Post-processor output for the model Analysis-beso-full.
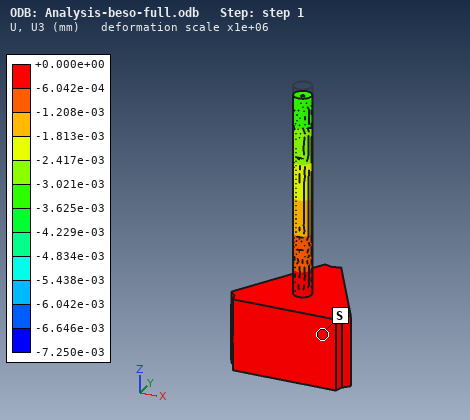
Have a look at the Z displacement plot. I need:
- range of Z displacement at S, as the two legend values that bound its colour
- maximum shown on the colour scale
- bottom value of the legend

-6.042e-04 to +0.000e+00 mm
+0.000e+00 mm
-7.250e-03 mm
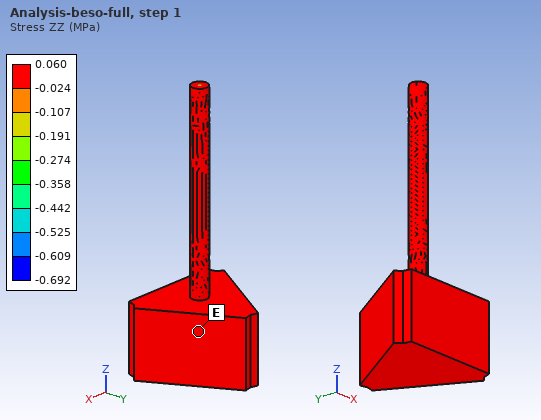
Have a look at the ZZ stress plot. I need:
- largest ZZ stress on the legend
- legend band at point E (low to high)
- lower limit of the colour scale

0.060 MPa
-0.024 to 0.060 MPa
-0.692 MPa
